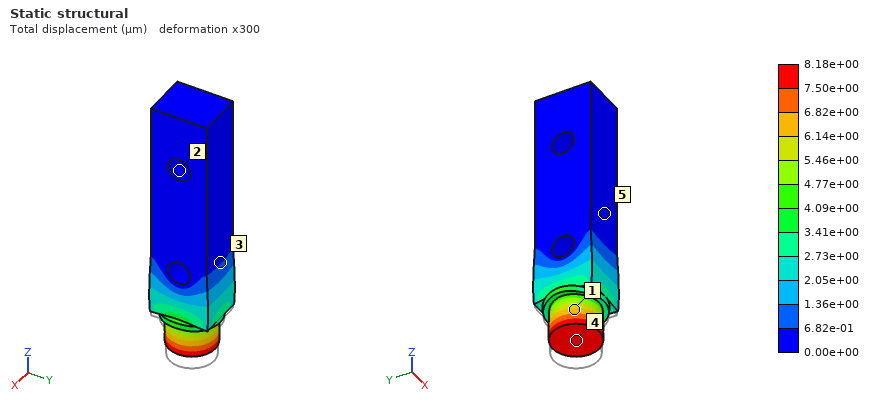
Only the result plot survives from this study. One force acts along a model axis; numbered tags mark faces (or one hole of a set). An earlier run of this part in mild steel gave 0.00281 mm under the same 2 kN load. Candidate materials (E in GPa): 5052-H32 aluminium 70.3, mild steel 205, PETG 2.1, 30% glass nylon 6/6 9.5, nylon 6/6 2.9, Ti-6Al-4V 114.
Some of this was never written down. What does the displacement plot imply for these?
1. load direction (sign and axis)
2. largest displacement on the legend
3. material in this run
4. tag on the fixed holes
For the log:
+Z
8.18e+00 µm
5052-H32 aluminium
2
